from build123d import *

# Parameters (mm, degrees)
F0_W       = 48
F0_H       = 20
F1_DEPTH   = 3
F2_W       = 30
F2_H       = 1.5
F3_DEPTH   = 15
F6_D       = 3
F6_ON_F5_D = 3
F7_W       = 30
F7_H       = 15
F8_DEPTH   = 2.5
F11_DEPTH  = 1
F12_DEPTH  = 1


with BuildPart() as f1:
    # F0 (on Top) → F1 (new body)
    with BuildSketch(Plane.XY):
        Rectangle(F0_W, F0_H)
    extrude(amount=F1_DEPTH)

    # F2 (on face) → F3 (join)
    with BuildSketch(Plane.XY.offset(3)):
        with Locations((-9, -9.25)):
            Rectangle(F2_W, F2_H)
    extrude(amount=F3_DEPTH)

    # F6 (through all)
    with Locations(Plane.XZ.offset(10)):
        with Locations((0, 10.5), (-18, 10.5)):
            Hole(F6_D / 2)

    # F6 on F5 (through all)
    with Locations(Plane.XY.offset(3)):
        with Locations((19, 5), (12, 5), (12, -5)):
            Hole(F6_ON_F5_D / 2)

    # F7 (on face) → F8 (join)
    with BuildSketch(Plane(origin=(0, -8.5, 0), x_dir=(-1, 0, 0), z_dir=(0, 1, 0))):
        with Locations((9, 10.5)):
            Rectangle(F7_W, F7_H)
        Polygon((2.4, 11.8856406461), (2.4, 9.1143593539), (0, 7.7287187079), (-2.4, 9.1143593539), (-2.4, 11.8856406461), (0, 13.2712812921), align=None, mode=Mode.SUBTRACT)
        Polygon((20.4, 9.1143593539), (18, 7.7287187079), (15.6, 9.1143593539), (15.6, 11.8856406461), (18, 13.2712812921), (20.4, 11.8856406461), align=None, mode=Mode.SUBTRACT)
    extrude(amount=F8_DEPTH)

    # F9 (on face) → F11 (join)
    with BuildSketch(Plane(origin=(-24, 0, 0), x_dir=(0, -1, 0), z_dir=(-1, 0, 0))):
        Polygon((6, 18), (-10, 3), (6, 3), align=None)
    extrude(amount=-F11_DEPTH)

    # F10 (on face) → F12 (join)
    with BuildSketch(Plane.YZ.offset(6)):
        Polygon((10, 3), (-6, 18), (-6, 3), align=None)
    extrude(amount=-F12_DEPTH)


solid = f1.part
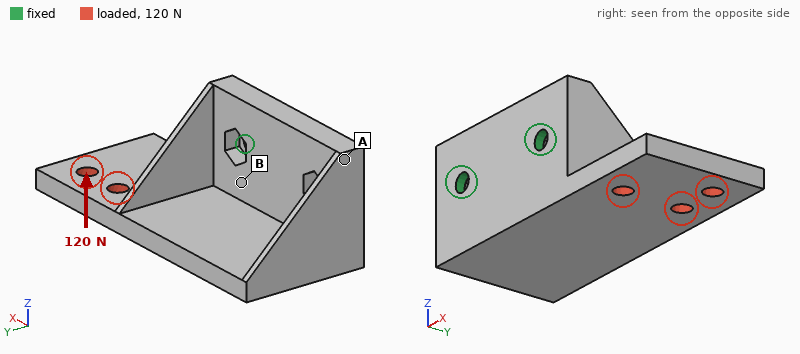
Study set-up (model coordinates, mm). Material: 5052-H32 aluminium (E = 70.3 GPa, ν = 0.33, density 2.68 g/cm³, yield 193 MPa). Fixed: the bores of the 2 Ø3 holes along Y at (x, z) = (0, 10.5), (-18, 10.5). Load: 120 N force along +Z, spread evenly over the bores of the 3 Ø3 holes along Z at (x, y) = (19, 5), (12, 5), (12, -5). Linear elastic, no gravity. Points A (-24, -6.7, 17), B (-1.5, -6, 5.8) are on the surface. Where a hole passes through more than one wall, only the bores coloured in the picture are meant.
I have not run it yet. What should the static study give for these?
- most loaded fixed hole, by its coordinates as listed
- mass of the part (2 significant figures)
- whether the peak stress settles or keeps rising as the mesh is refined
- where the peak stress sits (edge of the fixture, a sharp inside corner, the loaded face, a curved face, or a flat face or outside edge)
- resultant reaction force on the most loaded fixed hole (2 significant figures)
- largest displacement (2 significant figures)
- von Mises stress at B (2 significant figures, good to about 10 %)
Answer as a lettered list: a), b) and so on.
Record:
a) (0, 10.5)
b) 13 g
c) keeps rising
d) edge of the fixture
e) 210 N
f) 0.13 mm
g) 22 MPa
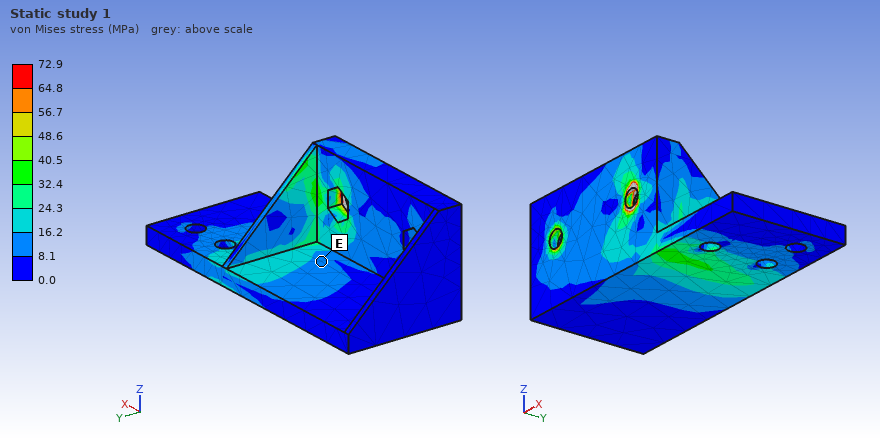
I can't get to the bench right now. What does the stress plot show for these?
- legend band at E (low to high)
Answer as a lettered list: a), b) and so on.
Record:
a) 8.1 to 16.2 MPa
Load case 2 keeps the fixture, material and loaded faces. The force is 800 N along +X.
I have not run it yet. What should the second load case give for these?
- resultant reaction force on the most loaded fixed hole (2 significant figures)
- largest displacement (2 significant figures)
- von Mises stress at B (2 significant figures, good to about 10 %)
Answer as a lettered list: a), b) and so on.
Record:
a) 720 N
b) 99 µm
c) 53 MPa
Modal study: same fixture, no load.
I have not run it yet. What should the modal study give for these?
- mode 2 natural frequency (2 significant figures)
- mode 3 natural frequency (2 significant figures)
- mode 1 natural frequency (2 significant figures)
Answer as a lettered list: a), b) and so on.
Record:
a) 5100 Hz
b) 6400 Hz
c) 3200 Hz
